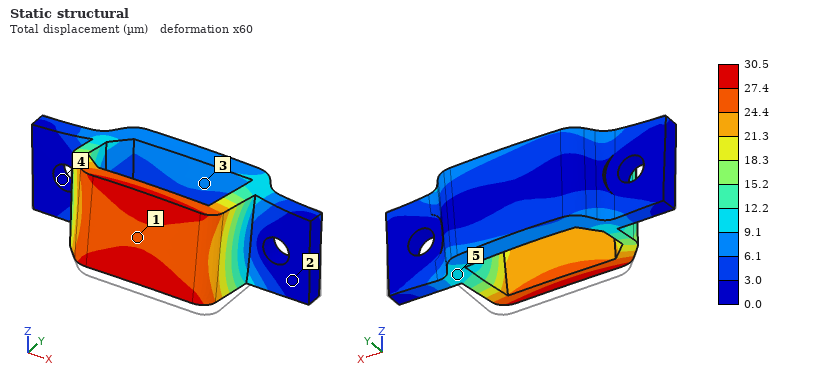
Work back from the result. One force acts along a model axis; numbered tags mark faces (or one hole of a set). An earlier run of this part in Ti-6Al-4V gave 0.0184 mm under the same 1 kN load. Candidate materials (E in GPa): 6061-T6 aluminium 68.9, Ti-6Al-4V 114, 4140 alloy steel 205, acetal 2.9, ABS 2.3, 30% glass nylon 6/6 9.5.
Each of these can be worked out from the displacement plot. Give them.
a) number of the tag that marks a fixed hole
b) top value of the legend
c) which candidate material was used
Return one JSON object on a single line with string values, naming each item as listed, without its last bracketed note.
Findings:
{"number of the tag that marks a fixed hole": "4", "top value of the legend": "30.5 µm", "which candidate material was used": "6061-T6 aluminium"}
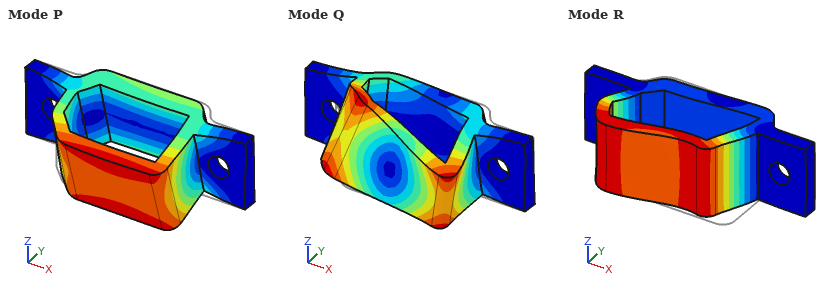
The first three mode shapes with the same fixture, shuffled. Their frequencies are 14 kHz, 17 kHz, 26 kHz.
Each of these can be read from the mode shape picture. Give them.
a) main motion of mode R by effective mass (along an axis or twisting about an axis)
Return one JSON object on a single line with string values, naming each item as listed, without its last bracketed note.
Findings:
{"main motion of mode R by effective mass": "along X"}
